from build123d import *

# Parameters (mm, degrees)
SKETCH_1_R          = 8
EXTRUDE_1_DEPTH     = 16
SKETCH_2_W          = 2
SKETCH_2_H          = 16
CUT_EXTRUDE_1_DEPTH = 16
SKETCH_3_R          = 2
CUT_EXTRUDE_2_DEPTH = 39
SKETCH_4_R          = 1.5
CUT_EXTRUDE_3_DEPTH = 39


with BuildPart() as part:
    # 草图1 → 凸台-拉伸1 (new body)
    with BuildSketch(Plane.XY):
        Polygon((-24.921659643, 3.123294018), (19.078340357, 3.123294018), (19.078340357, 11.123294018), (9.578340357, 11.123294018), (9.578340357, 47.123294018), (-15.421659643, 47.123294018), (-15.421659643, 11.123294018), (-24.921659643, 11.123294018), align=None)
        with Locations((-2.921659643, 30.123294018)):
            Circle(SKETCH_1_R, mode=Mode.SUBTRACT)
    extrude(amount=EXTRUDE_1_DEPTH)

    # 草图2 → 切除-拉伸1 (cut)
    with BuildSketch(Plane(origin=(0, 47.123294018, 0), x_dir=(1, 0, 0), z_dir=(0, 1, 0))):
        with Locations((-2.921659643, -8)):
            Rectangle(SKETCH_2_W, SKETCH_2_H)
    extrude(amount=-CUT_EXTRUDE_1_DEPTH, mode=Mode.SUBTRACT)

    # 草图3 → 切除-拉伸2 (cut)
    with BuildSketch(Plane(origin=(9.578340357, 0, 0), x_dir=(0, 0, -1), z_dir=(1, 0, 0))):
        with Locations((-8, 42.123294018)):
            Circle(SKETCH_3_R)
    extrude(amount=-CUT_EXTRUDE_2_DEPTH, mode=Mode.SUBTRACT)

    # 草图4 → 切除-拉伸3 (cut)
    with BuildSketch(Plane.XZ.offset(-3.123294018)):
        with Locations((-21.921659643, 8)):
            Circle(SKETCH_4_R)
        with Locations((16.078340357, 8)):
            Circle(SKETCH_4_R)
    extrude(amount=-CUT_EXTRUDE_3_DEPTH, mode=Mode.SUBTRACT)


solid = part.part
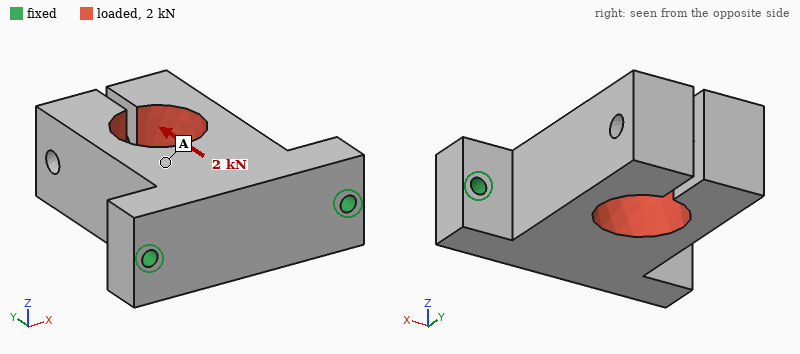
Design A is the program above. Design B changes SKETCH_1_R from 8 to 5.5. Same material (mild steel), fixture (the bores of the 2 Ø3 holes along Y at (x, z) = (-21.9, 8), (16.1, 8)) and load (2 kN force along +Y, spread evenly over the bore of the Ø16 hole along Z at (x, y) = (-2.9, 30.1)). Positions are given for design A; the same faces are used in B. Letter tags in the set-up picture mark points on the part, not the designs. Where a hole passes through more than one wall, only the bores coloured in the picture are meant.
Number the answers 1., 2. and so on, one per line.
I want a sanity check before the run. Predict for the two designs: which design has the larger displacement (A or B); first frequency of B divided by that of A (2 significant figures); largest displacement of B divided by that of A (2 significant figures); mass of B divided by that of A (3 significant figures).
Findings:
1. A
2. 0.96
3. 0.38
4. 1.10
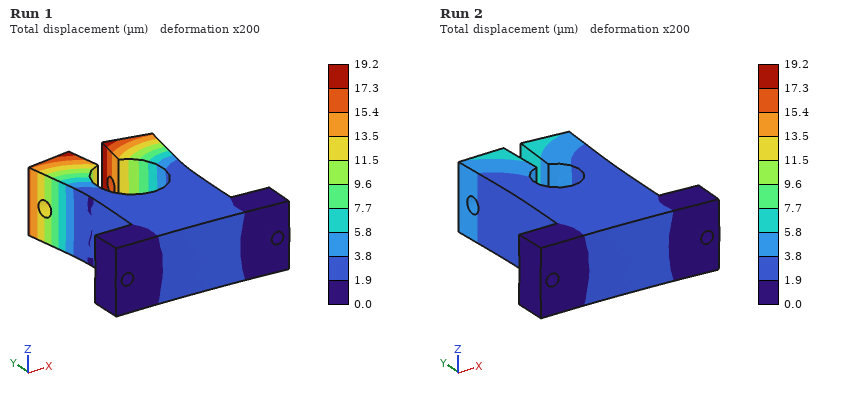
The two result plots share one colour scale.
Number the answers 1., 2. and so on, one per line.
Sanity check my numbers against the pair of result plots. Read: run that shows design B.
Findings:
1. Run 2
